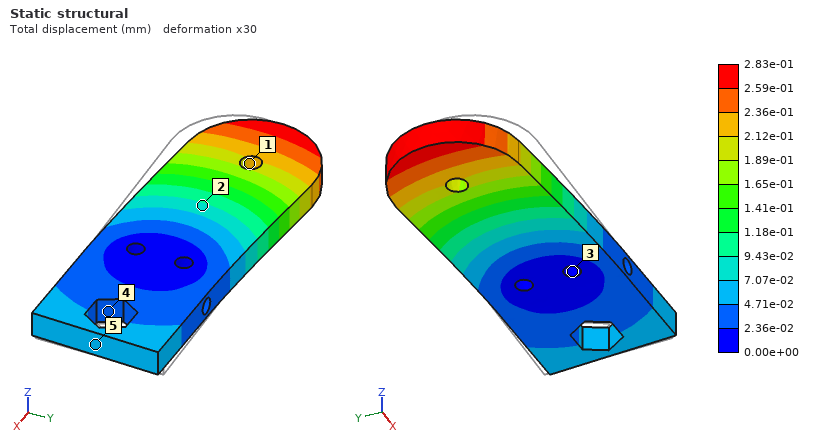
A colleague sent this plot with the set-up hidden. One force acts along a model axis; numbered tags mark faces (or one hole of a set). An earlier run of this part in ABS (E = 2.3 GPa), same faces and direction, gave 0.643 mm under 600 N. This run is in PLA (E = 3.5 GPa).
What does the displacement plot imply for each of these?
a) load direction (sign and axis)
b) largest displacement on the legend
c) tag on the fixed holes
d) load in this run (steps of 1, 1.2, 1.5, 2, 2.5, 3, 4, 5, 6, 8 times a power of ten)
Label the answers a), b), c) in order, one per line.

a) +Y
b) 2.83e-01 mm
c) 3
d) 400 N
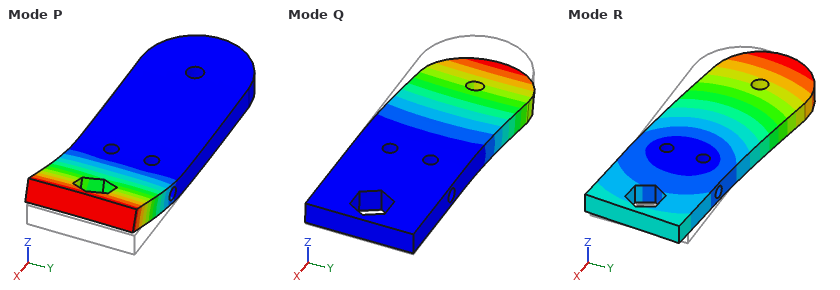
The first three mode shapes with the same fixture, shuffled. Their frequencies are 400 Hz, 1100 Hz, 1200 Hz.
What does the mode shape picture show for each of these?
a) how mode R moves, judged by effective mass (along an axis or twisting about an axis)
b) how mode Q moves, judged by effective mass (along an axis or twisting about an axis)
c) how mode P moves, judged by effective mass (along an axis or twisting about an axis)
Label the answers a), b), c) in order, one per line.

a) along Y
b) along Z
c) along Z
